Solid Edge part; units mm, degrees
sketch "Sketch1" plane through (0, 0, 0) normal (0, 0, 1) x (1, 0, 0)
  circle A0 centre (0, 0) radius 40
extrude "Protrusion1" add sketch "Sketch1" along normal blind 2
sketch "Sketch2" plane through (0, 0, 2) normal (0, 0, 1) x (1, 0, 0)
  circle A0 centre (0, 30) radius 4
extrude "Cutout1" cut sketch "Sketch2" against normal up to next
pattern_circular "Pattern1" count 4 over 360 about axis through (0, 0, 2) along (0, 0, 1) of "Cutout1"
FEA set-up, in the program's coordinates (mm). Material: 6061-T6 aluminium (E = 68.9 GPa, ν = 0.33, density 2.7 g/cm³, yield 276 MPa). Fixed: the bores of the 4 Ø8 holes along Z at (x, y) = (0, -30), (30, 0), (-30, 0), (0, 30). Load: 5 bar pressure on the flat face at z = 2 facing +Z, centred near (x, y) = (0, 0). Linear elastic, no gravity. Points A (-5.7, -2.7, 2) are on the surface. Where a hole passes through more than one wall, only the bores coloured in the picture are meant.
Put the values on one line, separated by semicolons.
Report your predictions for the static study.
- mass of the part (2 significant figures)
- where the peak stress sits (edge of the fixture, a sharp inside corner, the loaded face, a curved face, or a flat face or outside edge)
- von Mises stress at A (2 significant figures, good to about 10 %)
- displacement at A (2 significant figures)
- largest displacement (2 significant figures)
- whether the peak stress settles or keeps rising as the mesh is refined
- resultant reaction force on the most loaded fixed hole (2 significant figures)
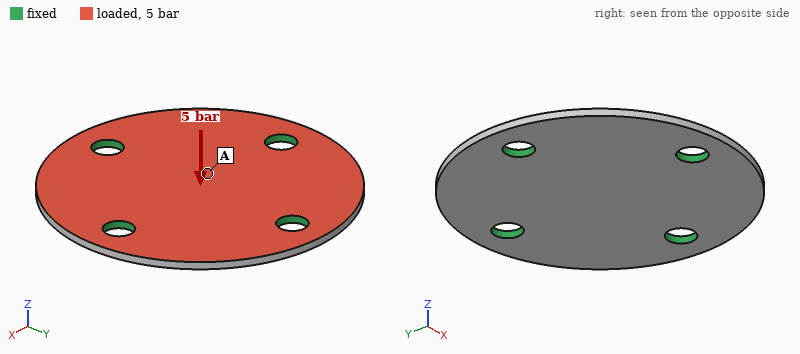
26 g; edge of the fixture; 37 MPa; 0.10 mm; 0.16 mm; keeps rising; 600 N
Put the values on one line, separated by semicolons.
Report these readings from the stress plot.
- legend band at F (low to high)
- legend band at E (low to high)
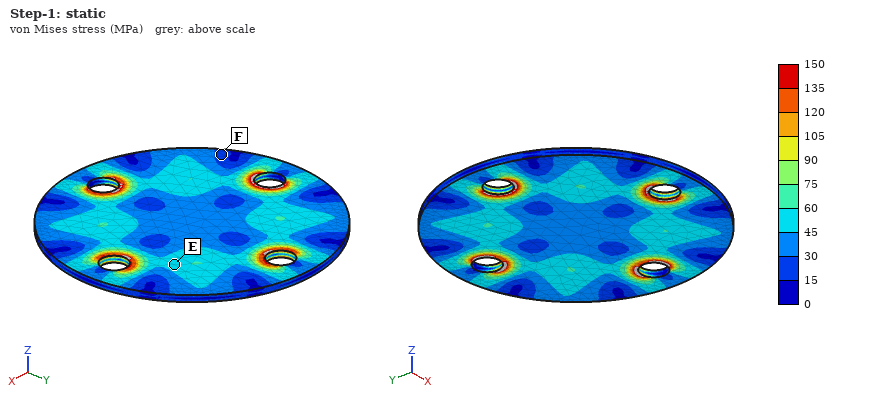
15 to 30 MPa; 45 to 60 MPa
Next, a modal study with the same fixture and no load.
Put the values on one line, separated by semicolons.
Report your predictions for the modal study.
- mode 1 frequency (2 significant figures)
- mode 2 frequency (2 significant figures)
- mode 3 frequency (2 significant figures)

4900 Hz; 5000 Hz; 5000 Hz
